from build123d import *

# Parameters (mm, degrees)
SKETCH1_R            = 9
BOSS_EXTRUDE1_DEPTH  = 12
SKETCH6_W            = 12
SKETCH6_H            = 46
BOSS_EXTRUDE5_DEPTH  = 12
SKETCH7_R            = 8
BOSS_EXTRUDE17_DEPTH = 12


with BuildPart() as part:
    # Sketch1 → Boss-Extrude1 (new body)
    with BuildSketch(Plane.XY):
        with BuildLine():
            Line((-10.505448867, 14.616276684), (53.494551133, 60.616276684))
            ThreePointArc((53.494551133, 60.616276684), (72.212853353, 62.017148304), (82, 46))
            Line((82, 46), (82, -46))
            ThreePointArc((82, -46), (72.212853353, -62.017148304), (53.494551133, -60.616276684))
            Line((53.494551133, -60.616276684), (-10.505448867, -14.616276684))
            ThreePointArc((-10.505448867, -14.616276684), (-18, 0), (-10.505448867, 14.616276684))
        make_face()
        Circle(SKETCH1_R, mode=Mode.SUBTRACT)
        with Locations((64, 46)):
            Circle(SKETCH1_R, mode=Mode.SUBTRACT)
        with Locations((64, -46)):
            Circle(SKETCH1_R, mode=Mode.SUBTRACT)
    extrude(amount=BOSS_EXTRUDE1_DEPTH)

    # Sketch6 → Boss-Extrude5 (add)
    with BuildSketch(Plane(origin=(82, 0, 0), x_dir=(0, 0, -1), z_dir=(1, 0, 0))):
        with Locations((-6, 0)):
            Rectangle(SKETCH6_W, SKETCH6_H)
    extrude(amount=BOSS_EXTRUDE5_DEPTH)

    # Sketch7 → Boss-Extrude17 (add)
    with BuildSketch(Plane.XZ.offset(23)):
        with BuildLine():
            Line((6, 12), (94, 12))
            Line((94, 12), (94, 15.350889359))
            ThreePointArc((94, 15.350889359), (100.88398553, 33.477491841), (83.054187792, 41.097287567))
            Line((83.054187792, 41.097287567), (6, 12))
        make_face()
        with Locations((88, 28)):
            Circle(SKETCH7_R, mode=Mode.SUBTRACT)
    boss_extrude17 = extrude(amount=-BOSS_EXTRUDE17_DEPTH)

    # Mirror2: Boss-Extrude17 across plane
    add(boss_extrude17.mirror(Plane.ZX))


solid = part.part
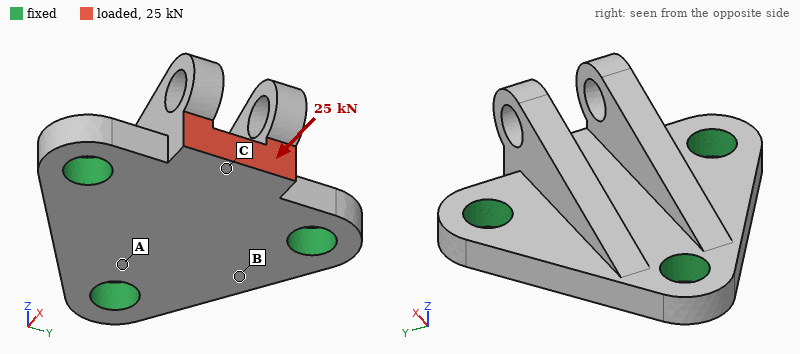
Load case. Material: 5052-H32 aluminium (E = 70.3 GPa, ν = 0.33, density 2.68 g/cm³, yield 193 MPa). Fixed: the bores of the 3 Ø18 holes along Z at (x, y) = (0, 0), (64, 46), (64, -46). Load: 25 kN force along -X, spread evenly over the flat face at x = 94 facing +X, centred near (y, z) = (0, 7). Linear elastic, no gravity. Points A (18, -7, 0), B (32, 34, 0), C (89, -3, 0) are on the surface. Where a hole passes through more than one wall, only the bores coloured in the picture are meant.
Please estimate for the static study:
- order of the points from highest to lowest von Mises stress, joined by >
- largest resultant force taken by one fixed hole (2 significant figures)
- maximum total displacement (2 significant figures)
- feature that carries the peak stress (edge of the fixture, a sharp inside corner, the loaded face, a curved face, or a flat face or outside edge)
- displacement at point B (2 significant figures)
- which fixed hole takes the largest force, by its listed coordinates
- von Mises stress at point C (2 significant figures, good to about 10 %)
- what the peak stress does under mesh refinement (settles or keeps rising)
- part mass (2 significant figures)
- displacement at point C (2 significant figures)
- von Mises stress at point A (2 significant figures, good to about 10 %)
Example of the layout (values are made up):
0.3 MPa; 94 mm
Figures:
C > A > B; 9.5 kN; 35 µm; a sharp inside corner; 6.7 µm; (0, 0); 34 MPa; keeps rising; 350 g; 32 µm; 21 MPa
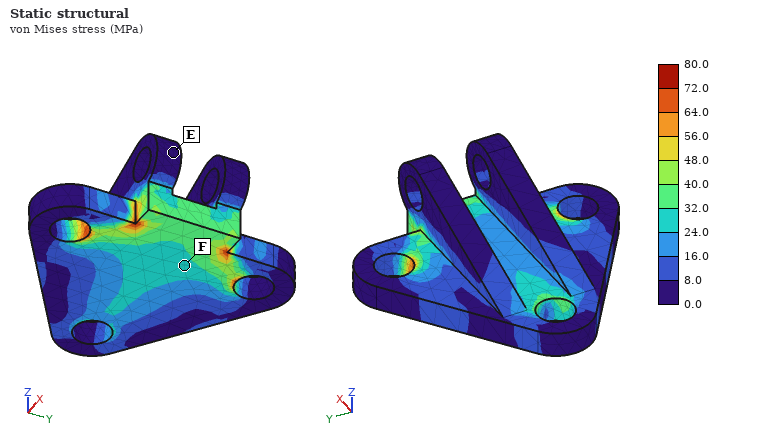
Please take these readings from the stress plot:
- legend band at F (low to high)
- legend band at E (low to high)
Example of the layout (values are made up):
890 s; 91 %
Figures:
24.0 to 32.0 MPa; 0.0 to 8.0 MPa
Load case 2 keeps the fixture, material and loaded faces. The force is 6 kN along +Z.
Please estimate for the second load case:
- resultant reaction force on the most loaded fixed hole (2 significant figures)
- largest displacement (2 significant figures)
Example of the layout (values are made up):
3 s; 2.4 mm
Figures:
4.1 kN; 0.11 mm
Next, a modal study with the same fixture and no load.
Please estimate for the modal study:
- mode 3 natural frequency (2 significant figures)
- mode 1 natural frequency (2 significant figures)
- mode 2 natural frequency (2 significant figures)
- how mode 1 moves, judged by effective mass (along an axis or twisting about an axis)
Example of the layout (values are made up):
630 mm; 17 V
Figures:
8400 Hz; 5100 Hz; 8100 Hz; along Z
